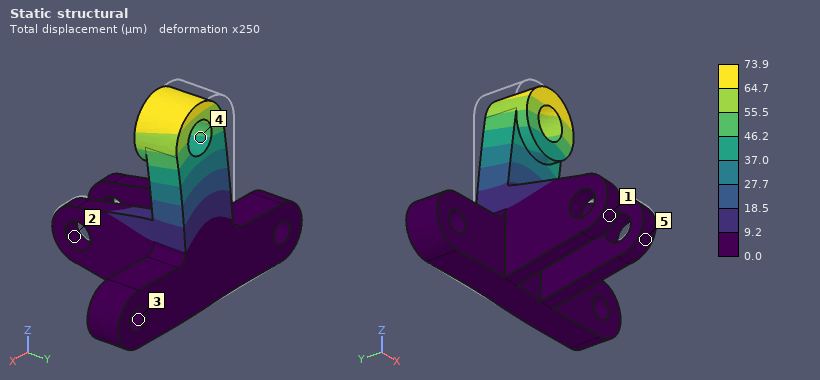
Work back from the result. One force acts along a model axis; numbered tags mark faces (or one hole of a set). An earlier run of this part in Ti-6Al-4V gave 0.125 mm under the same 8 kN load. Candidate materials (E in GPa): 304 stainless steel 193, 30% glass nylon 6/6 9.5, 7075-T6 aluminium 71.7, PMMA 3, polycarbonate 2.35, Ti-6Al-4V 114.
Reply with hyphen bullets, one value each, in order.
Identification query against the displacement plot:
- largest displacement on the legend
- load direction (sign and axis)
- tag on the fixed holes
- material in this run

- 73.9 µm
- +X
- 3
- 304 stainless steel
